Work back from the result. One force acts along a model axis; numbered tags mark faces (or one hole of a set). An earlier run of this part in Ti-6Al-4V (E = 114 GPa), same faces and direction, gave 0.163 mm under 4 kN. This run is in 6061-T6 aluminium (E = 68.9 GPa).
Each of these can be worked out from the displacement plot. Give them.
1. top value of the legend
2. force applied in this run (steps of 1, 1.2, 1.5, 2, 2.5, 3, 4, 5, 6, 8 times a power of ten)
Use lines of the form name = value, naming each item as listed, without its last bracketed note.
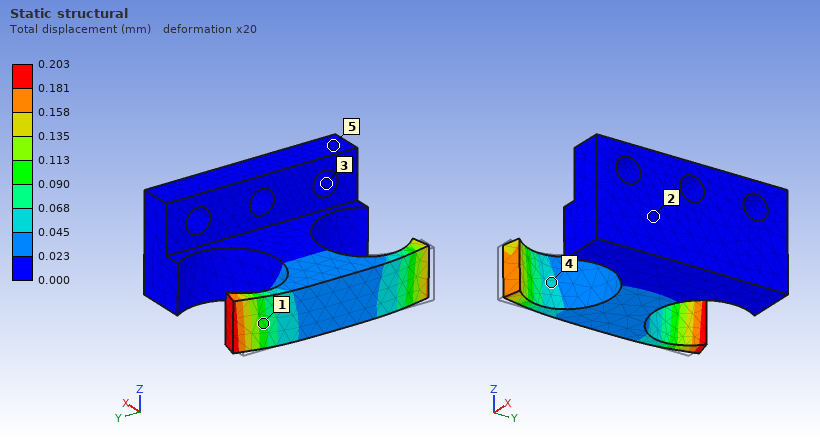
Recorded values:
top value of the legend = 0.203 mm
force applied in this run = 3 kN
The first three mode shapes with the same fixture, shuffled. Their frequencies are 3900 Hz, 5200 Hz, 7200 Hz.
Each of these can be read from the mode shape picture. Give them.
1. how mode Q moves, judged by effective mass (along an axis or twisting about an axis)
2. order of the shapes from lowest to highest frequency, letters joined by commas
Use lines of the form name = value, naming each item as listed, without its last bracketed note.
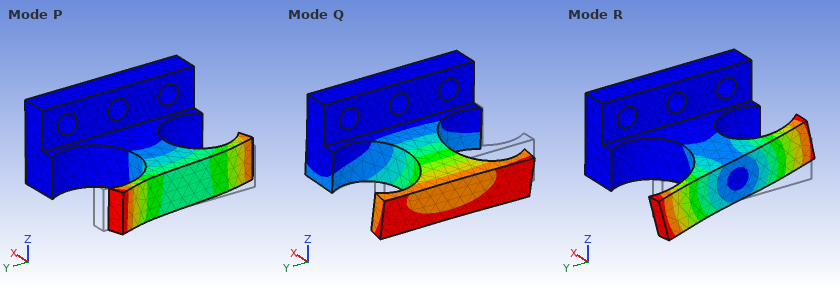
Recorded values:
how mode Q moves, judged by effective mass = along Z
order of the shapes from lowest to highest frequency, letters joined by commas = Q, P, R
